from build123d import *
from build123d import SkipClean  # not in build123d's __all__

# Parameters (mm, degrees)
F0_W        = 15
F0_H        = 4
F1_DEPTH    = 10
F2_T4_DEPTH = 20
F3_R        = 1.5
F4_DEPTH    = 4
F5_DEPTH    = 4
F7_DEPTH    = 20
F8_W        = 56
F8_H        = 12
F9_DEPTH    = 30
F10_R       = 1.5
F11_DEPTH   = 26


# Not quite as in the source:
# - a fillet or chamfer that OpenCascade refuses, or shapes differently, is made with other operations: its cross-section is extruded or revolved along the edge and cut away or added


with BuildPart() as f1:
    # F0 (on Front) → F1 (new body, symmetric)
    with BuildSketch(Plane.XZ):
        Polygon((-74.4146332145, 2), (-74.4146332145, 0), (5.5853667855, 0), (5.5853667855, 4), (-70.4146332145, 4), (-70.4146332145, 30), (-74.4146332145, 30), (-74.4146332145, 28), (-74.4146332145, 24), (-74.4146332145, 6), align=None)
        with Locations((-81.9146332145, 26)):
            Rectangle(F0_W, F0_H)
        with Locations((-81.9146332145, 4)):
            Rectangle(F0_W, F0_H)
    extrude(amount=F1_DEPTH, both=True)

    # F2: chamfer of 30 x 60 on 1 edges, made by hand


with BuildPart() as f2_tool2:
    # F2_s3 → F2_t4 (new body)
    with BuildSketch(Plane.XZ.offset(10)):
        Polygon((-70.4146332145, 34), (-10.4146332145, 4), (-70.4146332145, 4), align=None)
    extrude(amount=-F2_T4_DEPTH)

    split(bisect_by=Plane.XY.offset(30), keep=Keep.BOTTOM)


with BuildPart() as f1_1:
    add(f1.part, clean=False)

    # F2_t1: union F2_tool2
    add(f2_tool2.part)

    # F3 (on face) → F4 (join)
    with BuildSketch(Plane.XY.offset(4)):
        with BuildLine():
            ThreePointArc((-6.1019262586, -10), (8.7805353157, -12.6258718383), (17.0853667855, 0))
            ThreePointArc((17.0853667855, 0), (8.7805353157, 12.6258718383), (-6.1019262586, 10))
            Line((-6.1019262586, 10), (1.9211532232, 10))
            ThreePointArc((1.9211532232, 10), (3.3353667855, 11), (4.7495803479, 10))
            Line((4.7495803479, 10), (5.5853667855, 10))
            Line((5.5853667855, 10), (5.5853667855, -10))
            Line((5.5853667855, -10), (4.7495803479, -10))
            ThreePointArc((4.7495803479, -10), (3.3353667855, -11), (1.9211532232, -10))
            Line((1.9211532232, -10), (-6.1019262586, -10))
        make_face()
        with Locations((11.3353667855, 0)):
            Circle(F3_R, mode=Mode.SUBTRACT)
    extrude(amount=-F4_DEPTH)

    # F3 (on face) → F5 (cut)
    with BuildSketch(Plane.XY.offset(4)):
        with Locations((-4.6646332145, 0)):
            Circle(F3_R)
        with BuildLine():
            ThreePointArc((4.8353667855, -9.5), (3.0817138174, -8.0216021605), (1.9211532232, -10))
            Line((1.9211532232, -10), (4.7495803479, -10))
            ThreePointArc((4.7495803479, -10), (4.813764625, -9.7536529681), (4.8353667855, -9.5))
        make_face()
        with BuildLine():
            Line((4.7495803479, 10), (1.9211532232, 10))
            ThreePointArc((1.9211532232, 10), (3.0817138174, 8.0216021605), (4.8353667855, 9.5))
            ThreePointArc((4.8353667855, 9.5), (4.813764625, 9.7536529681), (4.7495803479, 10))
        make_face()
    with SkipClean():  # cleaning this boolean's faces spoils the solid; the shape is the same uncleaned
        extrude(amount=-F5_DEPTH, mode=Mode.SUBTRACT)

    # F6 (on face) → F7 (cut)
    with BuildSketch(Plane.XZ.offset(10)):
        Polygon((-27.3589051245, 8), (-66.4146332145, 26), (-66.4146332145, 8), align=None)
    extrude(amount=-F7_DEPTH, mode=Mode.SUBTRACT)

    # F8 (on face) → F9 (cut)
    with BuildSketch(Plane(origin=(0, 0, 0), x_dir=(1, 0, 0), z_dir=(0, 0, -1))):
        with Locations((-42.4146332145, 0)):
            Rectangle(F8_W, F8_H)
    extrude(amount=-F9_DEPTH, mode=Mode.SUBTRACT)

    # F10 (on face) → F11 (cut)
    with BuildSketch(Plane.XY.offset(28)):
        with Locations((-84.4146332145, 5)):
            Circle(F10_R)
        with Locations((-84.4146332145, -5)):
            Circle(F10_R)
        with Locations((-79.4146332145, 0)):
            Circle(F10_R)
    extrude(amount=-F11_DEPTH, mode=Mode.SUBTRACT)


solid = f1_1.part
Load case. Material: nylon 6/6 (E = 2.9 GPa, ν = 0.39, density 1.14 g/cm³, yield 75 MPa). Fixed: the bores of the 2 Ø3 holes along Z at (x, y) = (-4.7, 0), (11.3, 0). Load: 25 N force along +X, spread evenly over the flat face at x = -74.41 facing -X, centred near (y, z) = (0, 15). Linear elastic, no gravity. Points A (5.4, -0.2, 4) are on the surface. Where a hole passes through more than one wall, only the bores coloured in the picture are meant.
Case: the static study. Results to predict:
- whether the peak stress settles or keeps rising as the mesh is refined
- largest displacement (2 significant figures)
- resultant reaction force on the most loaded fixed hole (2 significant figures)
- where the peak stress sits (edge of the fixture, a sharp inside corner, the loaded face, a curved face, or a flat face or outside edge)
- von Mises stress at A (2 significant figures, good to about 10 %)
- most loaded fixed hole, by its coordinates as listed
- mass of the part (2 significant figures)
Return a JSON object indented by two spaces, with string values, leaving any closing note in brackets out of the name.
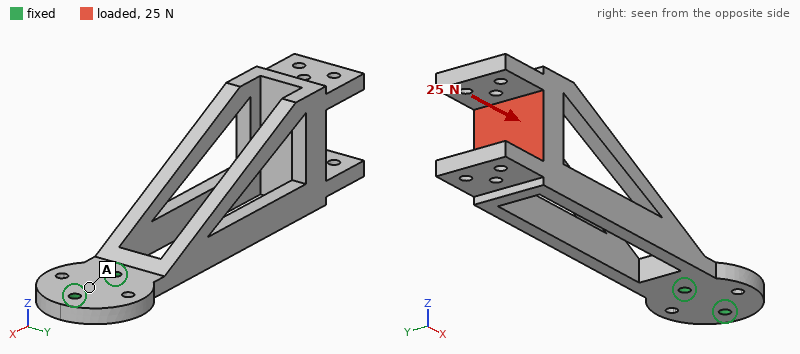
{
  "whether the peak stress settles or keeps rising as the mesh is refined": "keeps rising",
  "largest displacement": "1.3 mm",
  "resultant reaction force on the most loaded fixed hole": "20 N",
  "where the peak stress sits": "edge of the fixture",
  "von Mises stress at A": "0.89 MPa",
  "most loaded fixed hole, by its coordinates as listed": "(-4.7, 0)",
  "mass of the part": "15 g"
}
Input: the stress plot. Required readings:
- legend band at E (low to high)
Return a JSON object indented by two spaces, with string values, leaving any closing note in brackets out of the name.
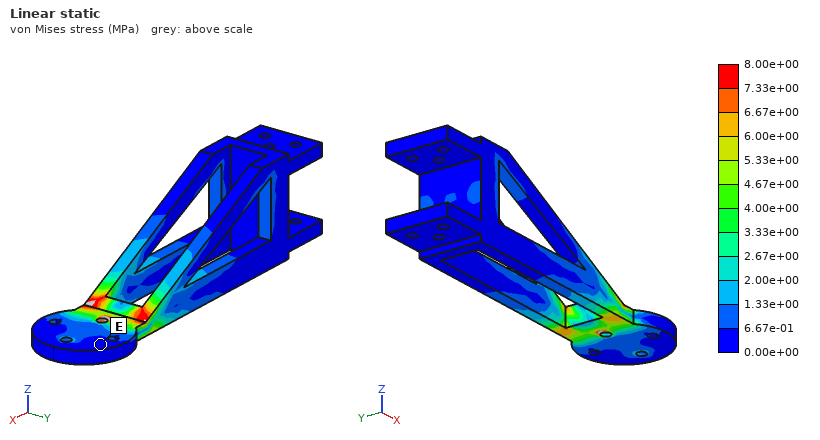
{
  "legend band at E": "0.00e+00 to 6.67e-01 MPa"
}
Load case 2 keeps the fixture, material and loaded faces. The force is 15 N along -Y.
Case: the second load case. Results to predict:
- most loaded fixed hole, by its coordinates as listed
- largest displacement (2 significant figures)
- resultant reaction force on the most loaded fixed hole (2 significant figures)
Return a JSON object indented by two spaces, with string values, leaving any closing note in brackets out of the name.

{
  "most loaded fixed hole, by its coordinates as listed": "(-4.7, 0)",
  "largest displacement": "1.3 mm",
  "resultant reaction force on the most loaded fixed hole": "68 N"
}
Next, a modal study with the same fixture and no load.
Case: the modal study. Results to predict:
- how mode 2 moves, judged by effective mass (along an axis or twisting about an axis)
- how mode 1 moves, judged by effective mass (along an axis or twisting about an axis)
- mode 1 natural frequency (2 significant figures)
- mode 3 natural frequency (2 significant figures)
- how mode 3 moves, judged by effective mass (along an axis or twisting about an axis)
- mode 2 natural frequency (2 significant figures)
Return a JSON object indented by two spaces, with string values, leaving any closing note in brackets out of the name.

{
  "how mode 2 moves, judged by effective mass": "along Y",
  "how mode 1 moves, judged by effective mass": "along Z",
  "mode 1 natural frequency": "120 Hz",
  "mode 3 natural frequency": "440 Hz",
  "how mode 3 moves, judged by effective mass": "twisting about X",
  "mode 2 natural frequency": "190 Hz"
}
